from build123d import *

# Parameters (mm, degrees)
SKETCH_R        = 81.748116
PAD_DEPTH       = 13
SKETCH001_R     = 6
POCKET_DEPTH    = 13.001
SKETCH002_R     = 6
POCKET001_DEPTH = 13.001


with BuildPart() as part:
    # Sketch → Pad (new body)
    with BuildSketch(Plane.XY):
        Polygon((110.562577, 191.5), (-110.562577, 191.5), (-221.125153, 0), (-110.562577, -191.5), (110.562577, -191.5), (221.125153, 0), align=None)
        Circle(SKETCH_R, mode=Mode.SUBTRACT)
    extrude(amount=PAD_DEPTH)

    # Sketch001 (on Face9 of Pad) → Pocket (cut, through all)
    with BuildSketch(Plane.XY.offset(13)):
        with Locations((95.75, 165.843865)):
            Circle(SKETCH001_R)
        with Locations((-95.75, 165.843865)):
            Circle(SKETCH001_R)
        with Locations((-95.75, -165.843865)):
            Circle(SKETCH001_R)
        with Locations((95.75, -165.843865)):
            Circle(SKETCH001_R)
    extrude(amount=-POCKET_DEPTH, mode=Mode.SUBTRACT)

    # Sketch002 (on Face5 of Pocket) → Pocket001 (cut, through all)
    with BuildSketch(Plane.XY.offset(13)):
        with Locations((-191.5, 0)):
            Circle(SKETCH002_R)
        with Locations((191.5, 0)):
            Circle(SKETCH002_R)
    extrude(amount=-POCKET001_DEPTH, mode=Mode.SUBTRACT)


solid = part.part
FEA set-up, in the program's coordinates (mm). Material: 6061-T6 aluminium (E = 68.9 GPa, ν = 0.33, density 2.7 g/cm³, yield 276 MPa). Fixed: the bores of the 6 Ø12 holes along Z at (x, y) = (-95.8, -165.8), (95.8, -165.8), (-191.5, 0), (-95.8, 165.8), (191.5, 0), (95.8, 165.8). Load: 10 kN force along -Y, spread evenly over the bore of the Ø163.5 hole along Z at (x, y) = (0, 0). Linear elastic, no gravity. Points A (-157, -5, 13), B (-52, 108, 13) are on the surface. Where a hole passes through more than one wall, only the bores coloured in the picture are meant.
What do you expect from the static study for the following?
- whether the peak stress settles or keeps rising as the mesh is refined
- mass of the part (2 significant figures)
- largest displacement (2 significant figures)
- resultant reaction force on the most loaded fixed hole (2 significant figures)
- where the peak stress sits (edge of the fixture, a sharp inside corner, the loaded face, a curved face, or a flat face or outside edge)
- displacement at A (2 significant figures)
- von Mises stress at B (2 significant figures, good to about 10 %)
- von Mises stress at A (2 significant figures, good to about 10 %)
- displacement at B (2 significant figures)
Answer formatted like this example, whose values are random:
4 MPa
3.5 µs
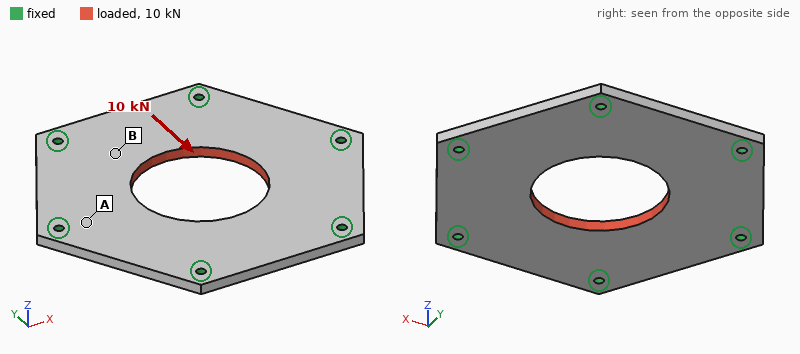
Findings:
keeps rising
3.7 kg
4.6 µm
2.1 kN
edge of the fixture
1.4 µm
1.8 MPa
0.63 MPa
3.2 µm
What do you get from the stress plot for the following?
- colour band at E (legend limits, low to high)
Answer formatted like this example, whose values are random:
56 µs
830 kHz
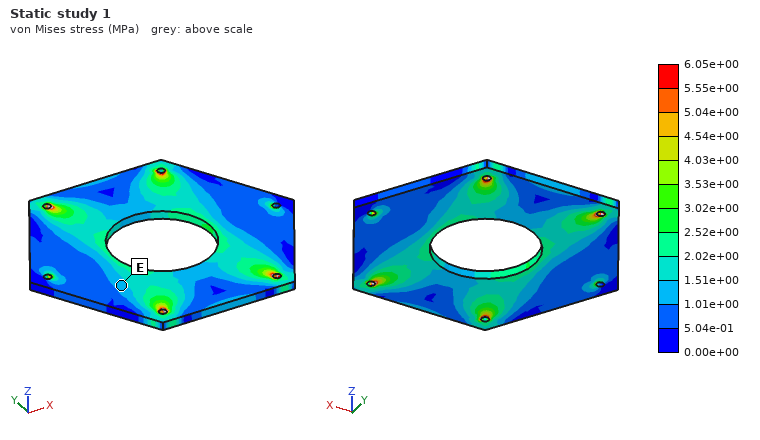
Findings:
1.01e+00 to 1.51e+00 MPa
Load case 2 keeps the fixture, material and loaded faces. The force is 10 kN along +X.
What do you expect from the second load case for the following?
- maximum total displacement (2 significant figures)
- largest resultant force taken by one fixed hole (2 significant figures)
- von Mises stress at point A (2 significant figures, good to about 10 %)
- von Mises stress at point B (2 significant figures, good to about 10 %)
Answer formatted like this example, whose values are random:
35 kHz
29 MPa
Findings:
4.5 µm
2.4 kN
3.3 MPa
1.4 MPa
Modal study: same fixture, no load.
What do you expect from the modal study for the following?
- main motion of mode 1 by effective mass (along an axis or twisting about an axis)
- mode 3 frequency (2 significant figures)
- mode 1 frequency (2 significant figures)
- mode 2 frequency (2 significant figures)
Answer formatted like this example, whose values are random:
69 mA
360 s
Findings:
along Z
1300 Hz
860 Hz
1300 Hz
